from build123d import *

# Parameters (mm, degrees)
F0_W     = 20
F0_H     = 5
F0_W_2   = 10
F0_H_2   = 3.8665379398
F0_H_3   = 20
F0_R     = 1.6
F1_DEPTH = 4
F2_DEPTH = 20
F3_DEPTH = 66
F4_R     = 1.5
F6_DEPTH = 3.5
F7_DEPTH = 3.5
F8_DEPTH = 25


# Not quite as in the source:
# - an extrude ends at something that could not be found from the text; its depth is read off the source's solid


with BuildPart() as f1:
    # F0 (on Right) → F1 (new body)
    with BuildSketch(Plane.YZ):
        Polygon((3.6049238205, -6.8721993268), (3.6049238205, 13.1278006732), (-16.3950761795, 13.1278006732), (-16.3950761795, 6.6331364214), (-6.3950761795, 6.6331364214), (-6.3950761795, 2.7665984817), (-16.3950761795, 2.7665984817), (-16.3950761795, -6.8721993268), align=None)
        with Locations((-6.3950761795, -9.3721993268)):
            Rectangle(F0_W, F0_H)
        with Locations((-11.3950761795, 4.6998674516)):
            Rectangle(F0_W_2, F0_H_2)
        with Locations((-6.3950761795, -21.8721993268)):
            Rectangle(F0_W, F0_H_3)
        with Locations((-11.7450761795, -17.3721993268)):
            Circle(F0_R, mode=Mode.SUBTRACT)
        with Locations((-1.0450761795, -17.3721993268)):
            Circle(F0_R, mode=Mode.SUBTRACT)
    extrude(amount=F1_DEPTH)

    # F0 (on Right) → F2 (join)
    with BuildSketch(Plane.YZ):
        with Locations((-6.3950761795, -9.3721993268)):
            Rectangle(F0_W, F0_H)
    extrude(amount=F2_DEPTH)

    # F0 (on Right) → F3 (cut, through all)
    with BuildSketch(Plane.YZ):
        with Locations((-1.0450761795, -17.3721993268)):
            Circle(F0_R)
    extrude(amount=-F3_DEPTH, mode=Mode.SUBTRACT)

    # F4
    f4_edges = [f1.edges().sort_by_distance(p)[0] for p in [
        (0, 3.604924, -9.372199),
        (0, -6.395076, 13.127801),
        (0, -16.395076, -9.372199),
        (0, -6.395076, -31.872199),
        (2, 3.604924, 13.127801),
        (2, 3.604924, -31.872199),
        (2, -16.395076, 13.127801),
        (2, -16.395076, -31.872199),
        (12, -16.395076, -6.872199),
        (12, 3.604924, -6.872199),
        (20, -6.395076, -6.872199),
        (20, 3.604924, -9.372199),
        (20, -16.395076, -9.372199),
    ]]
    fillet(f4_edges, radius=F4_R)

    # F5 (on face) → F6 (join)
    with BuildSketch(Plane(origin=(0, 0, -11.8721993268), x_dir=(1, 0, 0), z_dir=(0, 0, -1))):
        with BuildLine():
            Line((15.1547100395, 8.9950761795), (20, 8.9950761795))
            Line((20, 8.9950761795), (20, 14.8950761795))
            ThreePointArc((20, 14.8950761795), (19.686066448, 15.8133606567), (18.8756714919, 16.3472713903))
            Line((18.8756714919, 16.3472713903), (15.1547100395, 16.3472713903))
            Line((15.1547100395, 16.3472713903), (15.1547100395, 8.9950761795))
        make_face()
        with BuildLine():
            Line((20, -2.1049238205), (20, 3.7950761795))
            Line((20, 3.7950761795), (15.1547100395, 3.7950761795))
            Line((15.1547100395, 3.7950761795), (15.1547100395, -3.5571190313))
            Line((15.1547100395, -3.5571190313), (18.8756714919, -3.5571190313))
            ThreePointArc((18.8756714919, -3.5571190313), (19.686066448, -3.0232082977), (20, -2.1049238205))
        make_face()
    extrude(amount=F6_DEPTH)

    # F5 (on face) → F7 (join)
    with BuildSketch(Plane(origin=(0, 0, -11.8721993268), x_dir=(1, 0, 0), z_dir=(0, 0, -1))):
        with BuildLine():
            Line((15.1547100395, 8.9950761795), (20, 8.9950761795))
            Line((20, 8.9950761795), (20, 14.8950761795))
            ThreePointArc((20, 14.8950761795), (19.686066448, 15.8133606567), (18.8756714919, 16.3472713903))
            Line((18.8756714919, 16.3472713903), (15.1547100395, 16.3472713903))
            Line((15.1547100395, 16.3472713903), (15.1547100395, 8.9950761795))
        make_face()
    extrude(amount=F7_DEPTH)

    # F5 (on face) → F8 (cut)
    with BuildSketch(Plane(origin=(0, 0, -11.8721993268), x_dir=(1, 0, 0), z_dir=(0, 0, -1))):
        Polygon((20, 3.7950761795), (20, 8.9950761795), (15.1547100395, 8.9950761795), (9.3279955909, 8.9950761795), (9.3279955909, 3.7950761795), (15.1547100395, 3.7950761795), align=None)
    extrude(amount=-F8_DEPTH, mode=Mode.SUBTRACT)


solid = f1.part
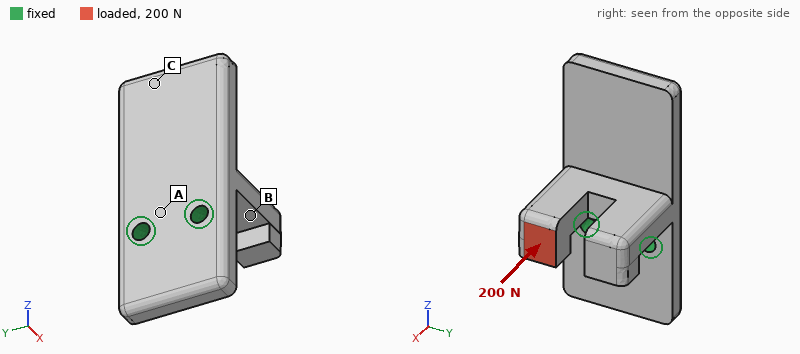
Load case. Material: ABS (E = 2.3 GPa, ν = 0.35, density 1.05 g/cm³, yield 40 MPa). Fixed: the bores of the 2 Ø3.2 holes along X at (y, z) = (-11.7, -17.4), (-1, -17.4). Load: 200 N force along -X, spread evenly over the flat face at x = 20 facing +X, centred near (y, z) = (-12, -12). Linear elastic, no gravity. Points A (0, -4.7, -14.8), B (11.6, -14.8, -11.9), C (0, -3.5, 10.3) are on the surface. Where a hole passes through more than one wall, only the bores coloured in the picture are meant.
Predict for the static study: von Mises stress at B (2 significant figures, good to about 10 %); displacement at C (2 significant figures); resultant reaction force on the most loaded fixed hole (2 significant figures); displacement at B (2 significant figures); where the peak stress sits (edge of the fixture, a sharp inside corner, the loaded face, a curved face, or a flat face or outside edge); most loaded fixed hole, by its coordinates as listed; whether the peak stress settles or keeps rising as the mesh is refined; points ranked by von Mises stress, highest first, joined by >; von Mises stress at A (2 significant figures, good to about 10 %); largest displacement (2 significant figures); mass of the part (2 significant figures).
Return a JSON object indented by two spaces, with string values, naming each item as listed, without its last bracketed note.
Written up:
{
  "von Mises stress at B": "19 MPa",
  "displacement at C": "0.24 mm",
  "resultant reaction force on the most loaded fixed hole": "180 N",
  "displacement at B": "0.18 mm",
  "where the peak stress sits": "edge of the fixture",
  "most loaded fixed hole, by its coordinates as listed": "(-11.7, -17.4)",
  "whether the peak stress settles or keeps rising as the mesh is refined": "keeps rising",
  "points ranked by von Mises stress, highest first, joined by >": "B > A > C",
  "von Mises stress at A": "7.5 MPa",
  "largest displacement": "0.36 mm",
  "mass of the part": "5.3 g"
}
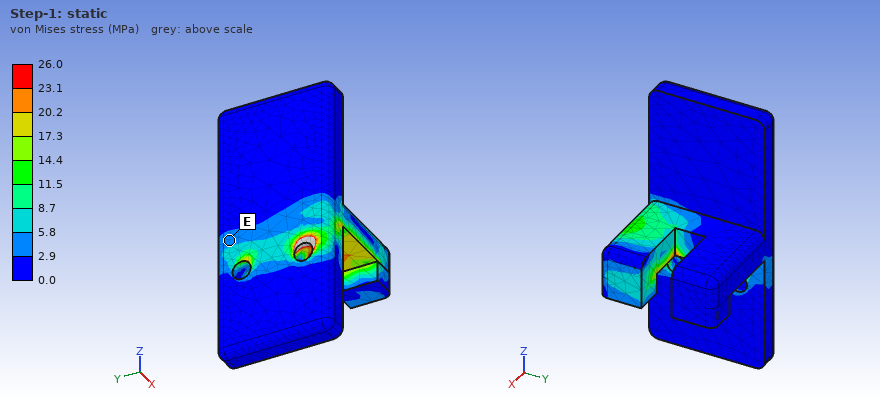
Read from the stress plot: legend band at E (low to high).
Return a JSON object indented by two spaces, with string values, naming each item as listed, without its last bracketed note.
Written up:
{
  "legend band at E": "2.9 to 5.8 MPa"
}
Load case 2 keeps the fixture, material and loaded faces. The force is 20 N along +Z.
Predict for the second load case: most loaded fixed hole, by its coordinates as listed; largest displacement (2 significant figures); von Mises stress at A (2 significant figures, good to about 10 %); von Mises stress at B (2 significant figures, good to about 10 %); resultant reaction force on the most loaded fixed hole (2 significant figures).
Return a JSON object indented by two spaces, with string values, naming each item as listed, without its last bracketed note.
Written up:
{
  "most loaded fixed hole, by its coordinates as listed": "(-11.7, -17.4)",
  "largest displacement": "0.35 mm",
  "von Mises stress at A": "4.7 MPa",
  "von Mises stress at B": "5.0 MPa",
  "resultant reaction force on the most loaded fixed hole": "19 N"
}
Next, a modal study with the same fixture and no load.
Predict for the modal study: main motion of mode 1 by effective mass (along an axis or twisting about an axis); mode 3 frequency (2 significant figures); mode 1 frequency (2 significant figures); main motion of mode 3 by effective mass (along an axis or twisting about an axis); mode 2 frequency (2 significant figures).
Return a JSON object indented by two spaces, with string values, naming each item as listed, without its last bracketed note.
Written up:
{
  "main motion of mode 1 by effective mass": "along X",
  "mode 3 frequency": "2900 Hz",
  "mode 1 frequency": "1000 Hz",
  "main motion of mode 3 by effective mass": "along Z",
  "mode 2 frequency": "2600 Hz"
}
